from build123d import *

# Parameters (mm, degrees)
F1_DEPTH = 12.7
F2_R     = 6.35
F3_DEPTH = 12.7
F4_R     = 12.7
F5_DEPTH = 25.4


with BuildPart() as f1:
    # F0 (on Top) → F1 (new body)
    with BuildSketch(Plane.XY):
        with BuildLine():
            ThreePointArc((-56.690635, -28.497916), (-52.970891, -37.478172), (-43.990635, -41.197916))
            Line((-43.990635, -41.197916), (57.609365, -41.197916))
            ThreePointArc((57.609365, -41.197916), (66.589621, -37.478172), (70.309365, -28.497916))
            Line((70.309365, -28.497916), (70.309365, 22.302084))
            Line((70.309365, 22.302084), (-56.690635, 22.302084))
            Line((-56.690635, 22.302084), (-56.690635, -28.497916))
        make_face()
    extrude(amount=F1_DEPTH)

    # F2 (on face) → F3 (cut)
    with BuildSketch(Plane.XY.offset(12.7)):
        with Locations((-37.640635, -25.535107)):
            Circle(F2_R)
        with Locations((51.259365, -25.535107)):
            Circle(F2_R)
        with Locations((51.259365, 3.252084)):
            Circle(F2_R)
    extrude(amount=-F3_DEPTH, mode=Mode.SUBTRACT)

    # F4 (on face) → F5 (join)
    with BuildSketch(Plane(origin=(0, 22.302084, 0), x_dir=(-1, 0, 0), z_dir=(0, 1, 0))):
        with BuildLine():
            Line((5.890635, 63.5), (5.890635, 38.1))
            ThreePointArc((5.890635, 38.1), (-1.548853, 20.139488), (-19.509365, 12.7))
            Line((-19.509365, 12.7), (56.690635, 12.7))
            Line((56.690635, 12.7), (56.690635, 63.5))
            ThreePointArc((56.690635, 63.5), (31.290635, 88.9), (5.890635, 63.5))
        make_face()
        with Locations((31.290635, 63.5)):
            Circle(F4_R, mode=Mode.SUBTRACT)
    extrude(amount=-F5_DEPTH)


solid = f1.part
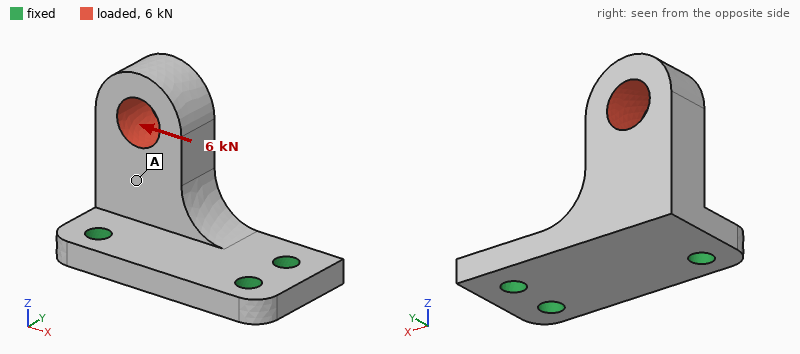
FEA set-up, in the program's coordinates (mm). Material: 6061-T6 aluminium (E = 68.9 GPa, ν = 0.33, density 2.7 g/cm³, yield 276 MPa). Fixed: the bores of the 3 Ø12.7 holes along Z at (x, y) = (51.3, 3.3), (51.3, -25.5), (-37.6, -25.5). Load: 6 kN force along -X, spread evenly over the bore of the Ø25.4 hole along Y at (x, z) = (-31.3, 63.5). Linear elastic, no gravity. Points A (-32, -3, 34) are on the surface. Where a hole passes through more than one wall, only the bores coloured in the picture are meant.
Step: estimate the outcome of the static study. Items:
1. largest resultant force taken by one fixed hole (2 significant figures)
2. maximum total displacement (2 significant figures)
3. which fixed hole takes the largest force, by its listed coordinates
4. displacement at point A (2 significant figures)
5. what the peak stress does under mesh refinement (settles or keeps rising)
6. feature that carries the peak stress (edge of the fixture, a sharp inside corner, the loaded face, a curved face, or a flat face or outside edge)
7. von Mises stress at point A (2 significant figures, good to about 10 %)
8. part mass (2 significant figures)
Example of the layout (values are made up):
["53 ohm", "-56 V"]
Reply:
["4.6 kN", "0.24 mm", "(-37.6, -25.5)", "0.079 mm", "keeps rising", "edge of the fixture", "19 MPa", "480 g"]
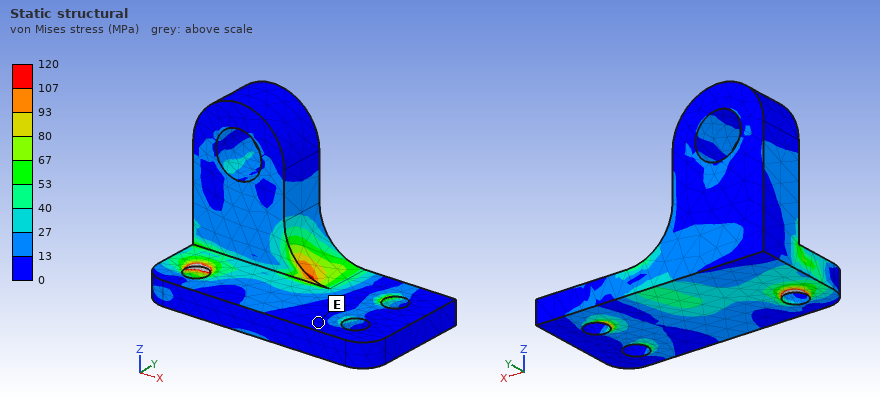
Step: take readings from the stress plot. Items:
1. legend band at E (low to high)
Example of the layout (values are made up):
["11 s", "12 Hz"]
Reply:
["0 to 13 MPa"]
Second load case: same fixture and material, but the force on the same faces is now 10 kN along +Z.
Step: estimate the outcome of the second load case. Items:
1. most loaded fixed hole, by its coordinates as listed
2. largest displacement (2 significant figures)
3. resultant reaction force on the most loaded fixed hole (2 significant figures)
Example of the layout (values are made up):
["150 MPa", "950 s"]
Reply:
["(-37.6, -25.5)", "0.45 mm", "8.4 kN"]
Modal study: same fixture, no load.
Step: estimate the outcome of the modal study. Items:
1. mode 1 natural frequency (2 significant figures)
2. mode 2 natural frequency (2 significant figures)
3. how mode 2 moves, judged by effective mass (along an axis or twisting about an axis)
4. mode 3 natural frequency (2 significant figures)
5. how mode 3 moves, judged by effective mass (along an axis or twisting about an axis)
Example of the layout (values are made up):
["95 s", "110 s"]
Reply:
["1300 Hz", "2700 Hz", "along X", "4600 Hz", "along Z"]
